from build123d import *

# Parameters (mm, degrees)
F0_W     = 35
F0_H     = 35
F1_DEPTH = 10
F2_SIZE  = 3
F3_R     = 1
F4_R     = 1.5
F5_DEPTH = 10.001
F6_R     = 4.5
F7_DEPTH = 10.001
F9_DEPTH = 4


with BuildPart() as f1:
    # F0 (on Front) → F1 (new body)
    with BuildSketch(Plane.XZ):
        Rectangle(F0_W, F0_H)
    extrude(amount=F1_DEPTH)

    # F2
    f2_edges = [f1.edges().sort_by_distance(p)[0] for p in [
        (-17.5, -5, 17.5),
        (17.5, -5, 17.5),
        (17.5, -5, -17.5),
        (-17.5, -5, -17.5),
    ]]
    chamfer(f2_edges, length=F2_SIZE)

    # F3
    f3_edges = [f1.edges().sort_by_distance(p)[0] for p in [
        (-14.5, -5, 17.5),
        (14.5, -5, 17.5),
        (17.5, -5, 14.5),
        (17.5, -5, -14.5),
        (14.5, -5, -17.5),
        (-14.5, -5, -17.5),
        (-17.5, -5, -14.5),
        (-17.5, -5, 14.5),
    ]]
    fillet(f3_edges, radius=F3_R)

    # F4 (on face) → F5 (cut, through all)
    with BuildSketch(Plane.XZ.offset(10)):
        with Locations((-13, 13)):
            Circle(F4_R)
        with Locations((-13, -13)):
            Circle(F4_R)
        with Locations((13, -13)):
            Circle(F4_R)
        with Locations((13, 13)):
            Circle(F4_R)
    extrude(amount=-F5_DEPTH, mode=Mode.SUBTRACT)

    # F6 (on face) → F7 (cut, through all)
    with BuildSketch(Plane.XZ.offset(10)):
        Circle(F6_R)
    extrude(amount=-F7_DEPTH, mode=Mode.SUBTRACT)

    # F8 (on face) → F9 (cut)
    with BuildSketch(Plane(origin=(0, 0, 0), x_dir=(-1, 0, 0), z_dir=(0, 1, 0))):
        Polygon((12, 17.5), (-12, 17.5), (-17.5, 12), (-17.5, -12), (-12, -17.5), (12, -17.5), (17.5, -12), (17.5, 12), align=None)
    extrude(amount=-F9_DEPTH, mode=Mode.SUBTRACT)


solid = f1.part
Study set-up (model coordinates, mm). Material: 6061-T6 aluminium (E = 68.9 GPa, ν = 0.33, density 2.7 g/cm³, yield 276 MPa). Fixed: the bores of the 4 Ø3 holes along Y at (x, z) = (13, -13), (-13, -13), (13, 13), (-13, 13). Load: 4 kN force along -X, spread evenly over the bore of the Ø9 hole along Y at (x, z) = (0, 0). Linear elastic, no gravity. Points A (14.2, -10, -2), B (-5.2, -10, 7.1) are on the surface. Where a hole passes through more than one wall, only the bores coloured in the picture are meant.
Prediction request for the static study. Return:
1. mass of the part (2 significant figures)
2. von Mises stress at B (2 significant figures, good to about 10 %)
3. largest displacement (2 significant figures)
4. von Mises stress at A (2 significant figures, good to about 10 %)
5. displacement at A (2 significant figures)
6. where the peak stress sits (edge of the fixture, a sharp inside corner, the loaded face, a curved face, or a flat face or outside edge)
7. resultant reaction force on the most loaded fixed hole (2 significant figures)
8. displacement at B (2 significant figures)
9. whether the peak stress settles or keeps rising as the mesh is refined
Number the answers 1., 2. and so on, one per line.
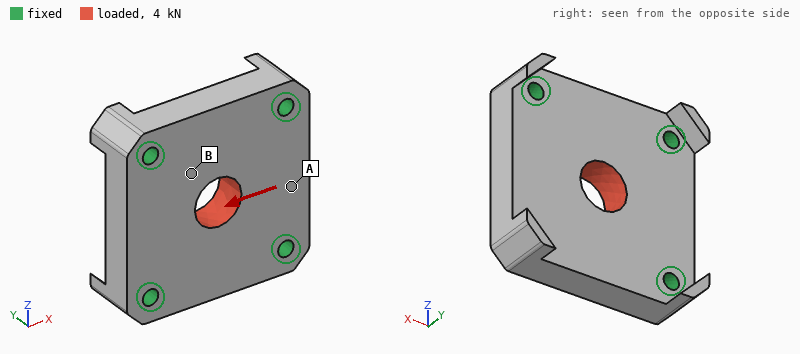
1. 19 g
2. 20 MPa
3. 6.1 µm
4. 7.2 MPa
5. 4.2 µm
6. edge of the fixture
7. 1.1 kN
8. 3.2 µm
9. keeps rising
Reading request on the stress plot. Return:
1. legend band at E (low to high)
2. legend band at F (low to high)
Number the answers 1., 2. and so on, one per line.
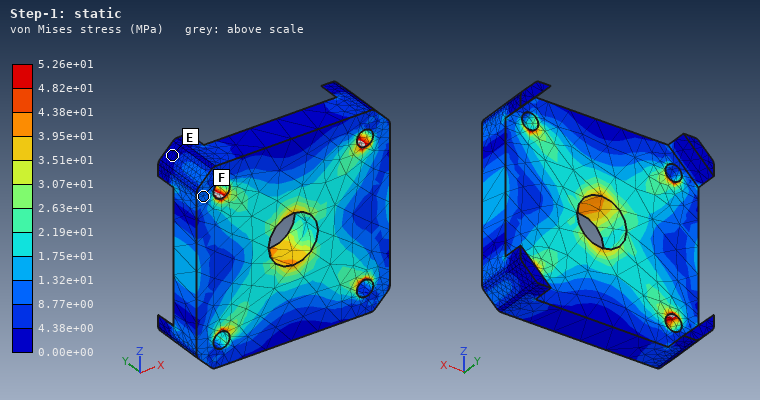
1. 0.00e+00 to 4.38e+00 MPa
2. 8.77e+00 to 1.32e+01 MPa
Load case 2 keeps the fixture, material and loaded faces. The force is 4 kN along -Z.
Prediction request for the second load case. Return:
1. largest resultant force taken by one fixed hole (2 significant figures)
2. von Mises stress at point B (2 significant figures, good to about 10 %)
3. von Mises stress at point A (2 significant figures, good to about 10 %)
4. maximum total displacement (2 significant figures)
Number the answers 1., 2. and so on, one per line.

1. 1.1 kN
2. 20 MPa
3. 5.3 MPa
4. 6.1 µm
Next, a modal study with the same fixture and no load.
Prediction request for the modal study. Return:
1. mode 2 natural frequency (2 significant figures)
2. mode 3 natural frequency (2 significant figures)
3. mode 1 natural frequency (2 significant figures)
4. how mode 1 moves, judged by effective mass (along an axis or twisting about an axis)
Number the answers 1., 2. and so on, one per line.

1. 38 kHz
2. 38 kHz
3. 27 kHz
4. along Y
